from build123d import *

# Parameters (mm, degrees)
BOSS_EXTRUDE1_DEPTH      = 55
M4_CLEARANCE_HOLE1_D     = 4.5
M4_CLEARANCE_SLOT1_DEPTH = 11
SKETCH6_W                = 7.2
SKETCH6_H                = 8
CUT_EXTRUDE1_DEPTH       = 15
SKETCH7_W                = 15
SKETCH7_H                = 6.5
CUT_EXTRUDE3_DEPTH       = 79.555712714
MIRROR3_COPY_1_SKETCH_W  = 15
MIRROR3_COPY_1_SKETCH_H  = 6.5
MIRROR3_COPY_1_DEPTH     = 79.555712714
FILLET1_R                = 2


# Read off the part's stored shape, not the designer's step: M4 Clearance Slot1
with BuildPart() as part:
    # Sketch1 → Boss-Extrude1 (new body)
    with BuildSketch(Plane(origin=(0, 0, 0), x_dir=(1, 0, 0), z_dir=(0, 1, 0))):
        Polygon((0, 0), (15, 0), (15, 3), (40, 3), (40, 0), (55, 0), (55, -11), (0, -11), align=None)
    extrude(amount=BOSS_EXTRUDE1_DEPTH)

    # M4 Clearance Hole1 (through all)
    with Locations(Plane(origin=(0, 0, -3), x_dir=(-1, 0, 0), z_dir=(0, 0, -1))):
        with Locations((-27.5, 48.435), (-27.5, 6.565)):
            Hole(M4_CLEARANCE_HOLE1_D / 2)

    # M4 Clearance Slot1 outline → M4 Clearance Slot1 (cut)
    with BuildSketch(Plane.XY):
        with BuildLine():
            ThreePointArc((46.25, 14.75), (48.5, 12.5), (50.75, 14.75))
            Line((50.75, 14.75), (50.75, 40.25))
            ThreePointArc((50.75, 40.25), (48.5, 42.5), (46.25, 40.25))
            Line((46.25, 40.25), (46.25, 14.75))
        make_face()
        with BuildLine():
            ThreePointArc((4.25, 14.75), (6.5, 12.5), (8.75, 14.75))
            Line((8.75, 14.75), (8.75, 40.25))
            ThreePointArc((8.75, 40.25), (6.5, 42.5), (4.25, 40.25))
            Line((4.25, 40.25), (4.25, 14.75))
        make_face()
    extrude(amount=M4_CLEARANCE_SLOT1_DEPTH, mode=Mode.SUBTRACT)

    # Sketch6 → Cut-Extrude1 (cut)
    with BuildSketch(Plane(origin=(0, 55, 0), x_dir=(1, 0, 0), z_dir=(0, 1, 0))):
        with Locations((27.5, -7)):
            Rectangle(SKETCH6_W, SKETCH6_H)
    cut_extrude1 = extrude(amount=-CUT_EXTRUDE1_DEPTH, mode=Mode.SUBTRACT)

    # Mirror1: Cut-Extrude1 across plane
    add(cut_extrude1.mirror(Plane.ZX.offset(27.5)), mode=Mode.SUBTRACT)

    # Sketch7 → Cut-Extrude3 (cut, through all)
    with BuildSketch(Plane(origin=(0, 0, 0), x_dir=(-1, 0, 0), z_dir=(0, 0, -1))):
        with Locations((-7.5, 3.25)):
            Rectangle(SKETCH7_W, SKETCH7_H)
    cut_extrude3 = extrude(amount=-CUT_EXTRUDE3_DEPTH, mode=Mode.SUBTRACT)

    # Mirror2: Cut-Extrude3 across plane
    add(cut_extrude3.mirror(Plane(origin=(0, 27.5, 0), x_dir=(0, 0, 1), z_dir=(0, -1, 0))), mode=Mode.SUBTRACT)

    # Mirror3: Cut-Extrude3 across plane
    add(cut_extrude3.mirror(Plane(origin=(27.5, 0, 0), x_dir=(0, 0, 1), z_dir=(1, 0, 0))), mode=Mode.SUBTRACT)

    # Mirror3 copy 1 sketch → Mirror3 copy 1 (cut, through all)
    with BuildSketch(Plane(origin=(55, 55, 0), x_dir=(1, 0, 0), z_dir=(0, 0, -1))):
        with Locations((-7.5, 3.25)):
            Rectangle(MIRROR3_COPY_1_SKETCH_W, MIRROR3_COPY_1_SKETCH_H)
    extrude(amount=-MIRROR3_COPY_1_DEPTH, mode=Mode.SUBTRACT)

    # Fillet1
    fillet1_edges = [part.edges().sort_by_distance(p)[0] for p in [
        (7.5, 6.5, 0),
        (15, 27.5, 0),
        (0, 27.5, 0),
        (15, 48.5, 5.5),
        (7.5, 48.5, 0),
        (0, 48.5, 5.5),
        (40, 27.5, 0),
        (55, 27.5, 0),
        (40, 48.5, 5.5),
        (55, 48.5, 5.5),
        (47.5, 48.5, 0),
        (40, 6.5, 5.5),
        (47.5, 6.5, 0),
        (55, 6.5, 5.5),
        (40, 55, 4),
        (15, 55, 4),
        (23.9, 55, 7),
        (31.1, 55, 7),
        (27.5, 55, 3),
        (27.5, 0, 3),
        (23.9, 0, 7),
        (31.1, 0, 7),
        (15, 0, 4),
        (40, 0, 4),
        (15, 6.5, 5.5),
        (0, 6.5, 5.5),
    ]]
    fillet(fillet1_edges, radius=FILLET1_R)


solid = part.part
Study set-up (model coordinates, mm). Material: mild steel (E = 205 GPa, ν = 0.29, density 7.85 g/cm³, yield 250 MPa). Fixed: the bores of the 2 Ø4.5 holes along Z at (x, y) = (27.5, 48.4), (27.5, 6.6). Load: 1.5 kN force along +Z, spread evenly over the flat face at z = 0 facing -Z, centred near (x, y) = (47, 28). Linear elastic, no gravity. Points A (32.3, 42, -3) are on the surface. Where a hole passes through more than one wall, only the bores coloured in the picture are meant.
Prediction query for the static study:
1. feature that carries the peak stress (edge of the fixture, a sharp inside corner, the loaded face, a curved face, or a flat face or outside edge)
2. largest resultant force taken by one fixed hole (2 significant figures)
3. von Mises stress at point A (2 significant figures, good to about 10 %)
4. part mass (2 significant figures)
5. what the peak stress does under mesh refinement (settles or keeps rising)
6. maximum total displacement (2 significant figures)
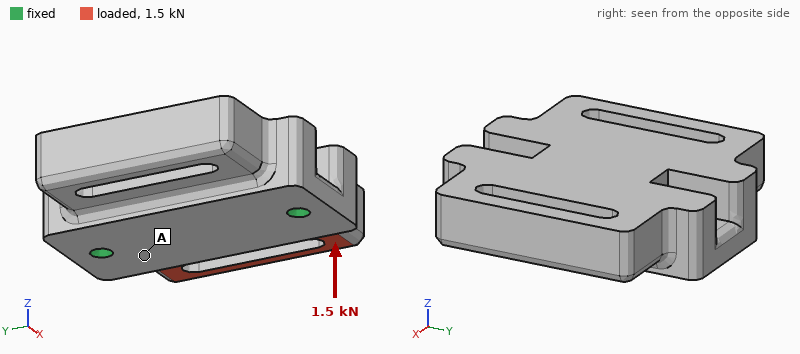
edge of the fixture
870 N
26 MPa
220 g
keeps rising
27 µm
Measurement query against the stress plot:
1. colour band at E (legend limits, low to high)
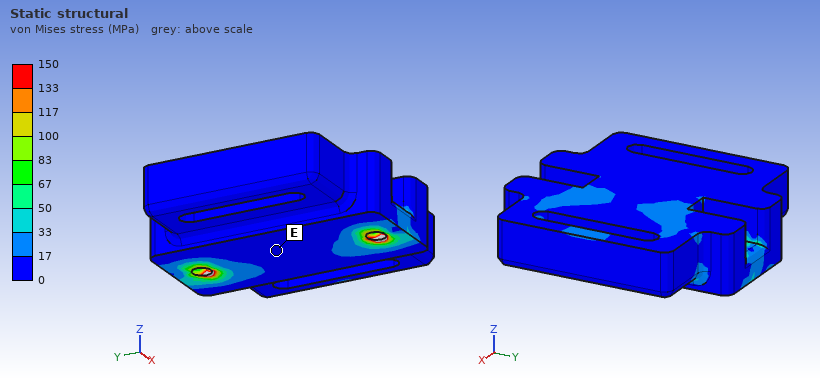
0 to 17 MPa
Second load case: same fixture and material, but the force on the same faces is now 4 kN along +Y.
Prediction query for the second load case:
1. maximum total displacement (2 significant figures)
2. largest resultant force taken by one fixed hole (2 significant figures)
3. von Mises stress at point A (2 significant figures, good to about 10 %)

13 µm
2.7 kN
34 MPa
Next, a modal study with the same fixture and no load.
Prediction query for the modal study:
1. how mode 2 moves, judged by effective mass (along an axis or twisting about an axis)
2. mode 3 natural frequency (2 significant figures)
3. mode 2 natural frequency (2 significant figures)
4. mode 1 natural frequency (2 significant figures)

along Z
15 kHz
10 kHz
4700 Hz
